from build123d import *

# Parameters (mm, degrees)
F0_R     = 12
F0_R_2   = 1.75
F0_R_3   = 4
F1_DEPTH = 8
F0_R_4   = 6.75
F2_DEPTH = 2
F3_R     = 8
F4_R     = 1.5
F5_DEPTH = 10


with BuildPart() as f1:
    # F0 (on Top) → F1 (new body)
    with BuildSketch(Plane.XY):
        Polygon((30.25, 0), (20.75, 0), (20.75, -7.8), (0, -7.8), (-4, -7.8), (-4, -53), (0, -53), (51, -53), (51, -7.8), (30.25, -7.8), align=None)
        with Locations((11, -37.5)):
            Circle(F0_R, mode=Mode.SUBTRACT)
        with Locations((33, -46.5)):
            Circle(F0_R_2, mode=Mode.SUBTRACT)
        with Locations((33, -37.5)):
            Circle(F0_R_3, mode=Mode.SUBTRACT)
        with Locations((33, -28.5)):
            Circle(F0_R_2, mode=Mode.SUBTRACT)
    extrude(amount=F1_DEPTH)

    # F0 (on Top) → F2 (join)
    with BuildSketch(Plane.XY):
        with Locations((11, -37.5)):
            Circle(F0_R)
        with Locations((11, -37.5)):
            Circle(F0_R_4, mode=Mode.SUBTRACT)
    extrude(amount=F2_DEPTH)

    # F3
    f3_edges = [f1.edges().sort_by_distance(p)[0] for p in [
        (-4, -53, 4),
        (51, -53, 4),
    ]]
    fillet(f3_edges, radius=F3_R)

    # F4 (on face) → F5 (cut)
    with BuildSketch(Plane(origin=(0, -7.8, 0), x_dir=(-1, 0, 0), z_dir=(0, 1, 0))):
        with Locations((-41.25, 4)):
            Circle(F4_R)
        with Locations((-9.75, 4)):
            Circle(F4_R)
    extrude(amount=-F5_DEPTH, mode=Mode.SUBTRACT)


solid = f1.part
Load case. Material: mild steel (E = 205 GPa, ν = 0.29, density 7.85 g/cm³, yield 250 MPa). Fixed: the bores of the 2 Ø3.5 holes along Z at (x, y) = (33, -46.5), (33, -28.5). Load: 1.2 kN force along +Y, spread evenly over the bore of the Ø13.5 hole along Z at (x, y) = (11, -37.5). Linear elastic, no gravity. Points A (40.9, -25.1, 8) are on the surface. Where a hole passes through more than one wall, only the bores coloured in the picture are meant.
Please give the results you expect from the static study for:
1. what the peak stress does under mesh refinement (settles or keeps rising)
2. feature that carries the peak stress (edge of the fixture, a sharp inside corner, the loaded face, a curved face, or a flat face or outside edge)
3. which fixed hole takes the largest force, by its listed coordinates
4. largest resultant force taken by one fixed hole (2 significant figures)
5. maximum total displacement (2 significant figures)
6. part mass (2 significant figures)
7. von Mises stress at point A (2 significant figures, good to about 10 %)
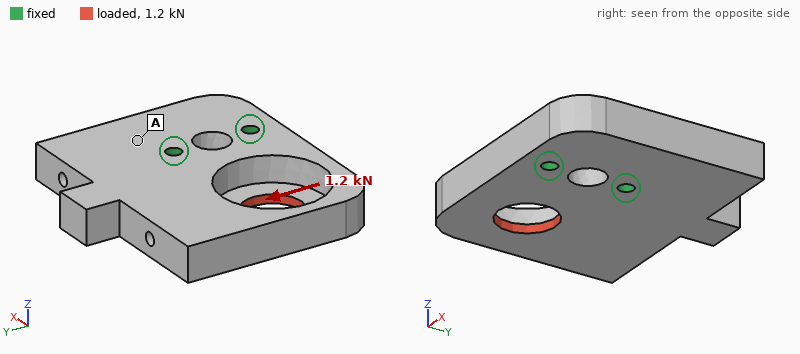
keeps rising
edge of the fixture
(33, -28.5)
1.4 kN
8.7 µm
130 g
7.9 MPa
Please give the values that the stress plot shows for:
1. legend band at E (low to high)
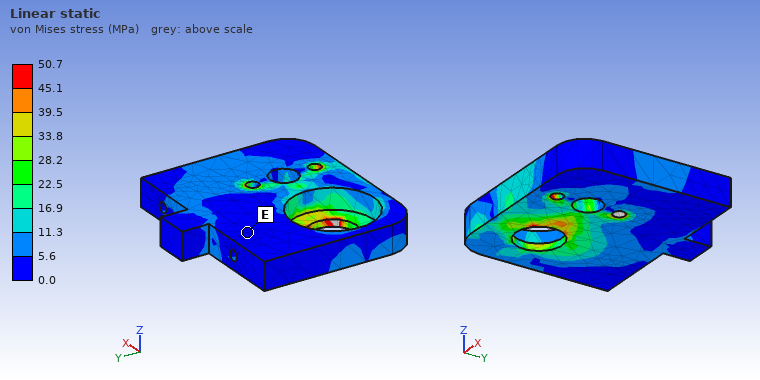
0.0 to 5.6 MPa
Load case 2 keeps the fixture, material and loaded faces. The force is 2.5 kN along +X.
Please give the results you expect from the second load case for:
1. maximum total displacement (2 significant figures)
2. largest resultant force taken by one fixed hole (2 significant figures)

16 µm
1.3 kN
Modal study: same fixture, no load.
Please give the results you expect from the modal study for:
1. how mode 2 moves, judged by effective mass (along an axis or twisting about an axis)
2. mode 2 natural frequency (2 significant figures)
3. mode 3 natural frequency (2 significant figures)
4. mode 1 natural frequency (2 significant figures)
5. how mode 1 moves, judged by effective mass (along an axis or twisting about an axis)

twisting about X
6700 Hz
8300 Hz
3900 Hz
along Z
